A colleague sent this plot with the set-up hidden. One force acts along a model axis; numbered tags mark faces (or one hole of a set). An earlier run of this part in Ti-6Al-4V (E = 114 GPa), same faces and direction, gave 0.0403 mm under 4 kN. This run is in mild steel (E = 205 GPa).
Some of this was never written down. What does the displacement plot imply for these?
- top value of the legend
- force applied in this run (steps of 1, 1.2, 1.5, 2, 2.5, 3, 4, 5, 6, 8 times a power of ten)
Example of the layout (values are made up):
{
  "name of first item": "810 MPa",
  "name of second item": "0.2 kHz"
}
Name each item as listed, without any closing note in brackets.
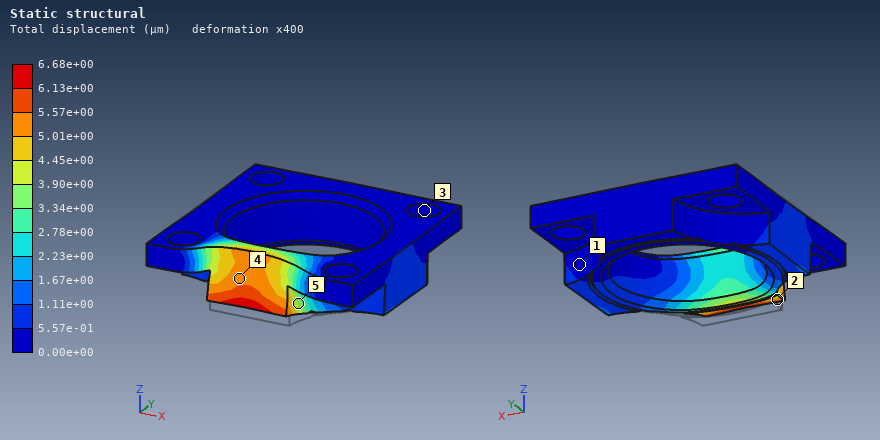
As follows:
{
  "top value of the legend": "6.68e+00 µm",
  "force applied in this run": "1.2 kN"
}
